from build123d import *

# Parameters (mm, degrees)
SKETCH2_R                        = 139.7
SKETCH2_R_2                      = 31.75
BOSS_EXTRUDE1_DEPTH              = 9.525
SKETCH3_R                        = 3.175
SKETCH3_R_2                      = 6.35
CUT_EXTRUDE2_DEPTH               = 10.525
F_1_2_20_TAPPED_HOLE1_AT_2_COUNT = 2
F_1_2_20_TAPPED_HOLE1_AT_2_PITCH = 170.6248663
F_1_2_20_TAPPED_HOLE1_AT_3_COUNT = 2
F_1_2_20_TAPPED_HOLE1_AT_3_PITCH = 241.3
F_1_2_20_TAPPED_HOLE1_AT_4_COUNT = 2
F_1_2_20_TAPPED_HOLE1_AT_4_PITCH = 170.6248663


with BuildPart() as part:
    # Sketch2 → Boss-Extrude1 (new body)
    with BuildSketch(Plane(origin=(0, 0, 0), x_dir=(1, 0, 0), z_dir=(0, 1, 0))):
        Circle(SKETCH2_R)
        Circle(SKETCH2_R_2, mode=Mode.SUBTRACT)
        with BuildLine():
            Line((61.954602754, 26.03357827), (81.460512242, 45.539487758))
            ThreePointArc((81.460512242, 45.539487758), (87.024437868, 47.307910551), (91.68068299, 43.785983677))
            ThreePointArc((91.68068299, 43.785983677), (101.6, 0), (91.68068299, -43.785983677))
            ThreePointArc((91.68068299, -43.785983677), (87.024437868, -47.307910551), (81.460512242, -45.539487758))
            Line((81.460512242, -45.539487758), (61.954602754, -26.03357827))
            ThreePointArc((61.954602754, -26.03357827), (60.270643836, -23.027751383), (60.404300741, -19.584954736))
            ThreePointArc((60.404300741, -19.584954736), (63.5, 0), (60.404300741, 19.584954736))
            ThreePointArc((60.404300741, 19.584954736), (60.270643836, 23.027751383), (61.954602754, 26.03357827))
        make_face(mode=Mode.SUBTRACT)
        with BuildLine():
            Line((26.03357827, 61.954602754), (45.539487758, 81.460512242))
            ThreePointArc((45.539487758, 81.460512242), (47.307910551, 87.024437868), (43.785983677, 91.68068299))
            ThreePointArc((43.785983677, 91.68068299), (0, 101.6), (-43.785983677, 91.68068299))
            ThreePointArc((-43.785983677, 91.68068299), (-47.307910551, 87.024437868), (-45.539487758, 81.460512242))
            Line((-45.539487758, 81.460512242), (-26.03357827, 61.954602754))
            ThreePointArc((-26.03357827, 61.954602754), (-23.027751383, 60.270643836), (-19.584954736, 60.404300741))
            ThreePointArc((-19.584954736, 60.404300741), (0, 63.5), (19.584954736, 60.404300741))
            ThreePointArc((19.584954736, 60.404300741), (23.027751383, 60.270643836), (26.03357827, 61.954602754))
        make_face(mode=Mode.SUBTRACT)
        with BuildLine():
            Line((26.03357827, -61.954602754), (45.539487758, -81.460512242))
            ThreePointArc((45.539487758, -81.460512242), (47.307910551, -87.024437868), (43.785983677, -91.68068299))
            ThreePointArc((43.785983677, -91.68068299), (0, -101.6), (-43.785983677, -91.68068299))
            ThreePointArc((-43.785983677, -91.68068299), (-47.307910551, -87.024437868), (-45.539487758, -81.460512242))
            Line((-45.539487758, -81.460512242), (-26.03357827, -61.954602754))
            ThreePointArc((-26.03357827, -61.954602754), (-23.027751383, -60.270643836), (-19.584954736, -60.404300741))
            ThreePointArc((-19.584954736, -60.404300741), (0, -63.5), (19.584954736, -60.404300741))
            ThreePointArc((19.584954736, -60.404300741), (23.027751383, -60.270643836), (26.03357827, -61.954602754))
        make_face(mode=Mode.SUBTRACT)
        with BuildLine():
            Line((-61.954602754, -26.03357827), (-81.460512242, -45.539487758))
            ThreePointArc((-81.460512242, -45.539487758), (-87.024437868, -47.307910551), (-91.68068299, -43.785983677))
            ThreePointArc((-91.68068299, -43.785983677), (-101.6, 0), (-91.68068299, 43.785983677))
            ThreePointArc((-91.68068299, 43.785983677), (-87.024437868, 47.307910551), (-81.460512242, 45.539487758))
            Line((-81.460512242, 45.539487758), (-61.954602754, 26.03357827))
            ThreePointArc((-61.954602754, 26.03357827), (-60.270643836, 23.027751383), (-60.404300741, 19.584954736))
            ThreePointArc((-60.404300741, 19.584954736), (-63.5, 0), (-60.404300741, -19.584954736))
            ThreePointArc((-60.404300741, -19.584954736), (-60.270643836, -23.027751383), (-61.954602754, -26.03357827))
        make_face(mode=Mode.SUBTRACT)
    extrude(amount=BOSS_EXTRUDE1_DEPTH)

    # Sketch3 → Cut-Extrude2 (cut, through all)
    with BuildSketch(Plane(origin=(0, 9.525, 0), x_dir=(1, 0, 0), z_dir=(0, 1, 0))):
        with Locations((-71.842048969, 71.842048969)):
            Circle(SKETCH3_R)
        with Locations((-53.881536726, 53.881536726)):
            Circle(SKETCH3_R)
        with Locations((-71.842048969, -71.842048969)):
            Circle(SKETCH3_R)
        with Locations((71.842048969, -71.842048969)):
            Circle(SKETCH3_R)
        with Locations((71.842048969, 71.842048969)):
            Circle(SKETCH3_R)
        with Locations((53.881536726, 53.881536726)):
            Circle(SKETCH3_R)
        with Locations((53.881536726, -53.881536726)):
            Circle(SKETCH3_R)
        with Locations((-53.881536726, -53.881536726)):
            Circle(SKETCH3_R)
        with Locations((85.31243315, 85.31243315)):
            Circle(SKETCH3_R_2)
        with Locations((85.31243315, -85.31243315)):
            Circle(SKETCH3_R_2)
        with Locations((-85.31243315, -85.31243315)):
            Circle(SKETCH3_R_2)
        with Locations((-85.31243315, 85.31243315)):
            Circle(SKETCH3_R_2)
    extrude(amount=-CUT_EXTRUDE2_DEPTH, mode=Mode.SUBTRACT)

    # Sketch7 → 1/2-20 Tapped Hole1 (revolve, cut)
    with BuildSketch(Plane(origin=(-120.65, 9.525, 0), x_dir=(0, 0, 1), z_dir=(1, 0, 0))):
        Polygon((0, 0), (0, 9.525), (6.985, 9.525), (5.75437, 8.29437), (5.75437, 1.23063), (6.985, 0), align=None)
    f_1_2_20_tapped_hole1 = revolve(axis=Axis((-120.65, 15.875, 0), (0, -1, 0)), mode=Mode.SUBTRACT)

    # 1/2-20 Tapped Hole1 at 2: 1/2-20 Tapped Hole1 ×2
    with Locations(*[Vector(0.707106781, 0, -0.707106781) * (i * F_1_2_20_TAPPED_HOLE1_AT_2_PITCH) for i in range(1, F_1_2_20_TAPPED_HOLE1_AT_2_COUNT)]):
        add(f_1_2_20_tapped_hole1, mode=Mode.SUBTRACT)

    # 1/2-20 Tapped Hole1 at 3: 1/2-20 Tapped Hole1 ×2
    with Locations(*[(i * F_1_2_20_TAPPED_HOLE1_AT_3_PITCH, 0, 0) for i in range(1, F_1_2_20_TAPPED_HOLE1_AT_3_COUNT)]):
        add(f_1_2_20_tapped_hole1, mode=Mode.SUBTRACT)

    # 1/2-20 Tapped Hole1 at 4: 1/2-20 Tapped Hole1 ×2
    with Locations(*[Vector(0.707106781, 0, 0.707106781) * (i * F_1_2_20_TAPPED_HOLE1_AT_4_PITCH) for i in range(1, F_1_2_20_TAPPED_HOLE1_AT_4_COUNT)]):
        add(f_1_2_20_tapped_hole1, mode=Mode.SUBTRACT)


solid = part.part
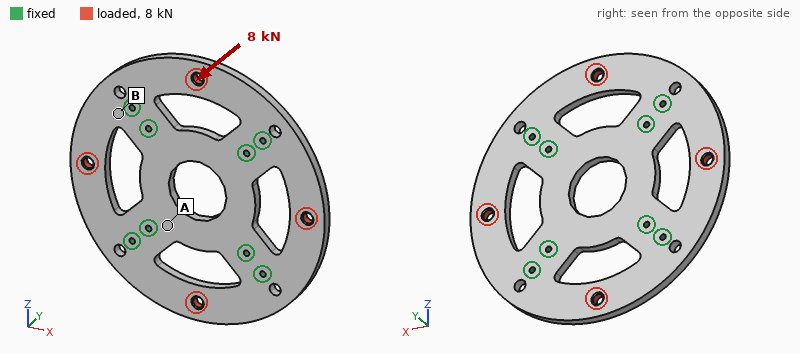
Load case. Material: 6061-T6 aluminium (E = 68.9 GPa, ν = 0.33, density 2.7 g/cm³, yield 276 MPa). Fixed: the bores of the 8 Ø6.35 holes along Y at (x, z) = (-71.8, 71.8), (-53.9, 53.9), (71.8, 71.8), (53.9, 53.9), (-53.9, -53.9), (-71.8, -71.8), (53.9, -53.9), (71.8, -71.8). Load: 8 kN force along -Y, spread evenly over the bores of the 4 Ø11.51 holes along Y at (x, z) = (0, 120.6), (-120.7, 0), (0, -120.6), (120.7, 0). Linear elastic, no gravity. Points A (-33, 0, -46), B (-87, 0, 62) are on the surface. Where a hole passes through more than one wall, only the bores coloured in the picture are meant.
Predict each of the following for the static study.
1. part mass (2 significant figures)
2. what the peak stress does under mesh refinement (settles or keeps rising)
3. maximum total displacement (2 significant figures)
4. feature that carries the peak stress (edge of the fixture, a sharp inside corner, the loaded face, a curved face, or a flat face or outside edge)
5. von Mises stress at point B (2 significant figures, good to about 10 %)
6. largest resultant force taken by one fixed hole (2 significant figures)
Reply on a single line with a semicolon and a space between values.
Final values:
1.2 kg; keeps rising; 0.51 mm; edge of the fixture; 53 MPa; 2.2 kN
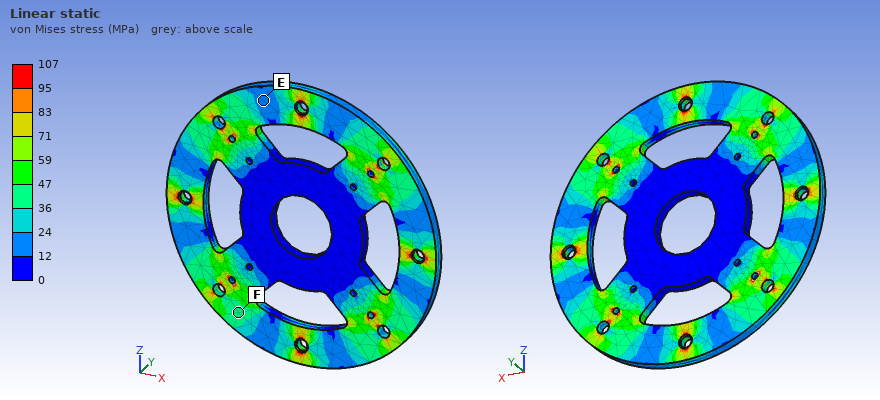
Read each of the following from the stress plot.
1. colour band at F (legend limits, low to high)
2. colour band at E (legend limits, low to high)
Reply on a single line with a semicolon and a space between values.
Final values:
36 to 47 MPa; 12 to 24 MPa
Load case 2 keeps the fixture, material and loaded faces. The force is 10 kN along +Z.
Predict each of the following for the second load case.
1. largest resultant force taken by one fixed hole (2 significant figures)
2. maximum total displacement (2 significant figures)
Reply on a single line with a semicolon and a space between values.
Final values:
2.4 kN; 18 µm
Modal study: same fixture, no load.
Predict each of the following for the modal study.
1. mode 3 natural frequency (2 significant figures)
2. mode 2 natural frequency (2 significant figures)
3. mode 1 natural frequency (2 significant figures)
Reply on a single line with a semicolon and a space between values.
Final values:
1200 Hz; 1200 Hz; 1100 Hz
